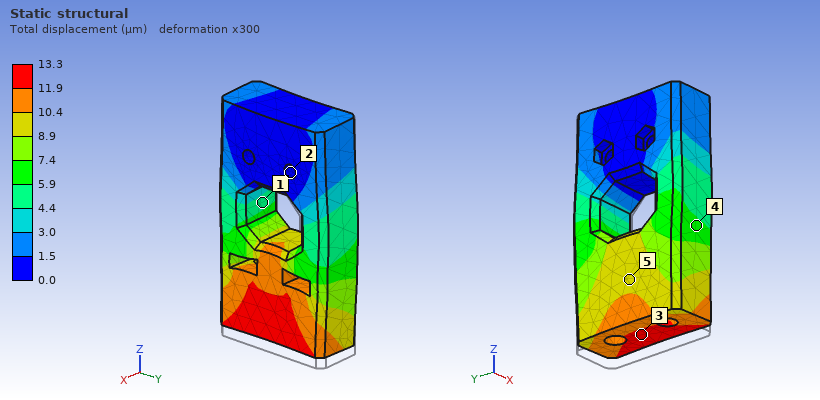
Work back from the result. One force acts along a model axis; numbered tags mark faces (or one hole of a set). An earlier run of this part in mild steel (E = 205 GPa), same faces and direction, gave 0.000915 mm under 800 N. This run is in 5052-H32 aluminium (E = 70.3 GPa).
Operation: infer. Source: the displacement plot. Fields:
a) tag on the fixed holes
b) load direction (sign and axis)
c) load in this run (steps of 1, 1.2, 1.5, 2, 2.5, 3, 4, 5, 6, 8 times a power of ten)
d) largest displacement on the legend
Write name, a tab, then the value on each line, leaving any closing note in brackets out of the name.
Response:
tag on the fixed holes	2
load direction	+Z
load in this run	4 kN
largest displacement on the legend	13.3 µm
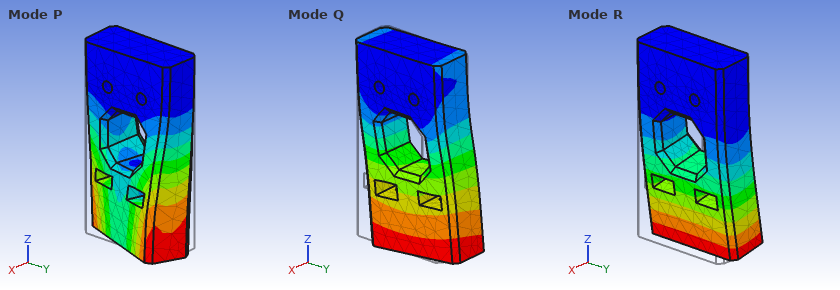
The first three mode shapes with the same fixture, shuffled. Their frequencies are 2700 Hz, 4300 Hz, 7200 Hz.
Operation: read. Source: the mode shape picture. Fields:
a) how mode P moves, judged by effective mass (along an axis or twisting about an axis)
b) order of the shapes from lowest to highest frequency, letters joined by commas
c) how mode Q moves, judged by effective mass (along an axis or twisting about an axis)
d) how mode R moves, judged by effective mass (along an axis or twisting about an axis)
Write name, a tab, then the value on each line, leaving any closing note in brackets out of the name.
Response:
how mode P moves, judged by effective mass	twisting about Z
order of the shapes from lowest to highest frequency, letters joined by commas	R, Q, P
how mode Q moves, judged by effective mass	along Y
how mode R moves, judged by effective mass	along X
